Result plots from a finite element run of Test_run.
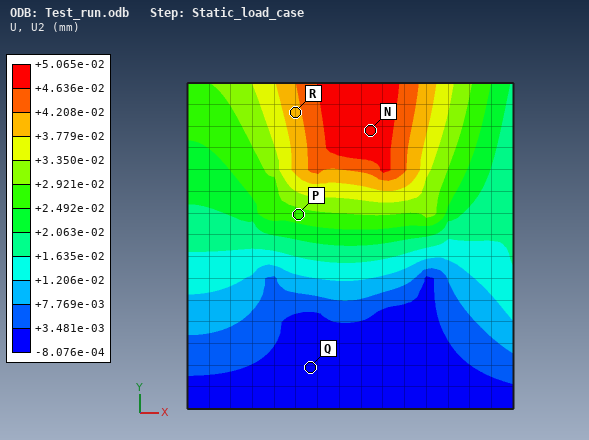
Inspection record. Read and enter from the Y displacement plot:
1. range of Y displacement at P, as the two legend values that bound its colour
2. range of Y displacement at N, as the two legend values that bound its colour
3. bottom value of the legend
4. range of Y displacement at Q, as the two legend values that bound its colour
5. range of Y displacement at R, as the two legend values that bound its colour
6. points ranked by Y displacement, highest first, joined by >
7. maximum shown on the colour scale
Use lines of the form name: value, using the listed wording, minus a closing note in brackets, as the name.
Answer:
range of Y displacement at P, as the two legend values that bound its colour: +2.492e-02 to +2.921e-02 mm
range of Y displacement at N, as the two legend values that bound its colour: +4.636e-02 to +5.065e-02 mm
bottom value of the legend: -8.076e-04 mm
range of Y displacement at Q, as the two legend values that bound its colour: -8.076e-04 to +3.481e-03 mm
range of Y displacement at R, as the two legend values that bound its colour: +3.779e-02 to +4.208e-02 mm
points ranked by Y displacement, highest first, joined by >: N > R > P > Q
maximum shown on the colour scale: +5.065e-02 mm
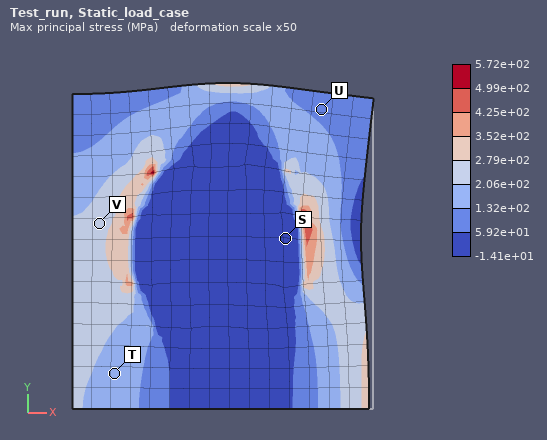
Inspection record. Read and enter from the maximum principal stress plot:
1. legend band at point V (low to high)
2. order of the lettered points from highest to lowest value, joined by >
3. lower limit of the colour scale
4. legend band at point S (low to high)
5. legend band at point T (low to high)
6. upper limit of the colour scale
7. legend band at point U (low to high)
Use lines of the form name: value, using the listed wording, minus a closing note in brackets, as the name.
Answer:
legend band at point V: 2.06e+02 to 2.79e+02 MPa
order of the lettered points from highest to lowest value, joined by >: V > T > U > S
lower limit of the colour scale: -1.41e+01 MPa
legend band at point S: -1.41e+01 to 5.92e+01 MPa
legend band at point T: 1.32e+02 to 2.06e+02 MPa
upper limit of the colour scale: 5.72e+02 MPa
legend band at point U: 5.92e+01 to 1.32e+02 MPa
